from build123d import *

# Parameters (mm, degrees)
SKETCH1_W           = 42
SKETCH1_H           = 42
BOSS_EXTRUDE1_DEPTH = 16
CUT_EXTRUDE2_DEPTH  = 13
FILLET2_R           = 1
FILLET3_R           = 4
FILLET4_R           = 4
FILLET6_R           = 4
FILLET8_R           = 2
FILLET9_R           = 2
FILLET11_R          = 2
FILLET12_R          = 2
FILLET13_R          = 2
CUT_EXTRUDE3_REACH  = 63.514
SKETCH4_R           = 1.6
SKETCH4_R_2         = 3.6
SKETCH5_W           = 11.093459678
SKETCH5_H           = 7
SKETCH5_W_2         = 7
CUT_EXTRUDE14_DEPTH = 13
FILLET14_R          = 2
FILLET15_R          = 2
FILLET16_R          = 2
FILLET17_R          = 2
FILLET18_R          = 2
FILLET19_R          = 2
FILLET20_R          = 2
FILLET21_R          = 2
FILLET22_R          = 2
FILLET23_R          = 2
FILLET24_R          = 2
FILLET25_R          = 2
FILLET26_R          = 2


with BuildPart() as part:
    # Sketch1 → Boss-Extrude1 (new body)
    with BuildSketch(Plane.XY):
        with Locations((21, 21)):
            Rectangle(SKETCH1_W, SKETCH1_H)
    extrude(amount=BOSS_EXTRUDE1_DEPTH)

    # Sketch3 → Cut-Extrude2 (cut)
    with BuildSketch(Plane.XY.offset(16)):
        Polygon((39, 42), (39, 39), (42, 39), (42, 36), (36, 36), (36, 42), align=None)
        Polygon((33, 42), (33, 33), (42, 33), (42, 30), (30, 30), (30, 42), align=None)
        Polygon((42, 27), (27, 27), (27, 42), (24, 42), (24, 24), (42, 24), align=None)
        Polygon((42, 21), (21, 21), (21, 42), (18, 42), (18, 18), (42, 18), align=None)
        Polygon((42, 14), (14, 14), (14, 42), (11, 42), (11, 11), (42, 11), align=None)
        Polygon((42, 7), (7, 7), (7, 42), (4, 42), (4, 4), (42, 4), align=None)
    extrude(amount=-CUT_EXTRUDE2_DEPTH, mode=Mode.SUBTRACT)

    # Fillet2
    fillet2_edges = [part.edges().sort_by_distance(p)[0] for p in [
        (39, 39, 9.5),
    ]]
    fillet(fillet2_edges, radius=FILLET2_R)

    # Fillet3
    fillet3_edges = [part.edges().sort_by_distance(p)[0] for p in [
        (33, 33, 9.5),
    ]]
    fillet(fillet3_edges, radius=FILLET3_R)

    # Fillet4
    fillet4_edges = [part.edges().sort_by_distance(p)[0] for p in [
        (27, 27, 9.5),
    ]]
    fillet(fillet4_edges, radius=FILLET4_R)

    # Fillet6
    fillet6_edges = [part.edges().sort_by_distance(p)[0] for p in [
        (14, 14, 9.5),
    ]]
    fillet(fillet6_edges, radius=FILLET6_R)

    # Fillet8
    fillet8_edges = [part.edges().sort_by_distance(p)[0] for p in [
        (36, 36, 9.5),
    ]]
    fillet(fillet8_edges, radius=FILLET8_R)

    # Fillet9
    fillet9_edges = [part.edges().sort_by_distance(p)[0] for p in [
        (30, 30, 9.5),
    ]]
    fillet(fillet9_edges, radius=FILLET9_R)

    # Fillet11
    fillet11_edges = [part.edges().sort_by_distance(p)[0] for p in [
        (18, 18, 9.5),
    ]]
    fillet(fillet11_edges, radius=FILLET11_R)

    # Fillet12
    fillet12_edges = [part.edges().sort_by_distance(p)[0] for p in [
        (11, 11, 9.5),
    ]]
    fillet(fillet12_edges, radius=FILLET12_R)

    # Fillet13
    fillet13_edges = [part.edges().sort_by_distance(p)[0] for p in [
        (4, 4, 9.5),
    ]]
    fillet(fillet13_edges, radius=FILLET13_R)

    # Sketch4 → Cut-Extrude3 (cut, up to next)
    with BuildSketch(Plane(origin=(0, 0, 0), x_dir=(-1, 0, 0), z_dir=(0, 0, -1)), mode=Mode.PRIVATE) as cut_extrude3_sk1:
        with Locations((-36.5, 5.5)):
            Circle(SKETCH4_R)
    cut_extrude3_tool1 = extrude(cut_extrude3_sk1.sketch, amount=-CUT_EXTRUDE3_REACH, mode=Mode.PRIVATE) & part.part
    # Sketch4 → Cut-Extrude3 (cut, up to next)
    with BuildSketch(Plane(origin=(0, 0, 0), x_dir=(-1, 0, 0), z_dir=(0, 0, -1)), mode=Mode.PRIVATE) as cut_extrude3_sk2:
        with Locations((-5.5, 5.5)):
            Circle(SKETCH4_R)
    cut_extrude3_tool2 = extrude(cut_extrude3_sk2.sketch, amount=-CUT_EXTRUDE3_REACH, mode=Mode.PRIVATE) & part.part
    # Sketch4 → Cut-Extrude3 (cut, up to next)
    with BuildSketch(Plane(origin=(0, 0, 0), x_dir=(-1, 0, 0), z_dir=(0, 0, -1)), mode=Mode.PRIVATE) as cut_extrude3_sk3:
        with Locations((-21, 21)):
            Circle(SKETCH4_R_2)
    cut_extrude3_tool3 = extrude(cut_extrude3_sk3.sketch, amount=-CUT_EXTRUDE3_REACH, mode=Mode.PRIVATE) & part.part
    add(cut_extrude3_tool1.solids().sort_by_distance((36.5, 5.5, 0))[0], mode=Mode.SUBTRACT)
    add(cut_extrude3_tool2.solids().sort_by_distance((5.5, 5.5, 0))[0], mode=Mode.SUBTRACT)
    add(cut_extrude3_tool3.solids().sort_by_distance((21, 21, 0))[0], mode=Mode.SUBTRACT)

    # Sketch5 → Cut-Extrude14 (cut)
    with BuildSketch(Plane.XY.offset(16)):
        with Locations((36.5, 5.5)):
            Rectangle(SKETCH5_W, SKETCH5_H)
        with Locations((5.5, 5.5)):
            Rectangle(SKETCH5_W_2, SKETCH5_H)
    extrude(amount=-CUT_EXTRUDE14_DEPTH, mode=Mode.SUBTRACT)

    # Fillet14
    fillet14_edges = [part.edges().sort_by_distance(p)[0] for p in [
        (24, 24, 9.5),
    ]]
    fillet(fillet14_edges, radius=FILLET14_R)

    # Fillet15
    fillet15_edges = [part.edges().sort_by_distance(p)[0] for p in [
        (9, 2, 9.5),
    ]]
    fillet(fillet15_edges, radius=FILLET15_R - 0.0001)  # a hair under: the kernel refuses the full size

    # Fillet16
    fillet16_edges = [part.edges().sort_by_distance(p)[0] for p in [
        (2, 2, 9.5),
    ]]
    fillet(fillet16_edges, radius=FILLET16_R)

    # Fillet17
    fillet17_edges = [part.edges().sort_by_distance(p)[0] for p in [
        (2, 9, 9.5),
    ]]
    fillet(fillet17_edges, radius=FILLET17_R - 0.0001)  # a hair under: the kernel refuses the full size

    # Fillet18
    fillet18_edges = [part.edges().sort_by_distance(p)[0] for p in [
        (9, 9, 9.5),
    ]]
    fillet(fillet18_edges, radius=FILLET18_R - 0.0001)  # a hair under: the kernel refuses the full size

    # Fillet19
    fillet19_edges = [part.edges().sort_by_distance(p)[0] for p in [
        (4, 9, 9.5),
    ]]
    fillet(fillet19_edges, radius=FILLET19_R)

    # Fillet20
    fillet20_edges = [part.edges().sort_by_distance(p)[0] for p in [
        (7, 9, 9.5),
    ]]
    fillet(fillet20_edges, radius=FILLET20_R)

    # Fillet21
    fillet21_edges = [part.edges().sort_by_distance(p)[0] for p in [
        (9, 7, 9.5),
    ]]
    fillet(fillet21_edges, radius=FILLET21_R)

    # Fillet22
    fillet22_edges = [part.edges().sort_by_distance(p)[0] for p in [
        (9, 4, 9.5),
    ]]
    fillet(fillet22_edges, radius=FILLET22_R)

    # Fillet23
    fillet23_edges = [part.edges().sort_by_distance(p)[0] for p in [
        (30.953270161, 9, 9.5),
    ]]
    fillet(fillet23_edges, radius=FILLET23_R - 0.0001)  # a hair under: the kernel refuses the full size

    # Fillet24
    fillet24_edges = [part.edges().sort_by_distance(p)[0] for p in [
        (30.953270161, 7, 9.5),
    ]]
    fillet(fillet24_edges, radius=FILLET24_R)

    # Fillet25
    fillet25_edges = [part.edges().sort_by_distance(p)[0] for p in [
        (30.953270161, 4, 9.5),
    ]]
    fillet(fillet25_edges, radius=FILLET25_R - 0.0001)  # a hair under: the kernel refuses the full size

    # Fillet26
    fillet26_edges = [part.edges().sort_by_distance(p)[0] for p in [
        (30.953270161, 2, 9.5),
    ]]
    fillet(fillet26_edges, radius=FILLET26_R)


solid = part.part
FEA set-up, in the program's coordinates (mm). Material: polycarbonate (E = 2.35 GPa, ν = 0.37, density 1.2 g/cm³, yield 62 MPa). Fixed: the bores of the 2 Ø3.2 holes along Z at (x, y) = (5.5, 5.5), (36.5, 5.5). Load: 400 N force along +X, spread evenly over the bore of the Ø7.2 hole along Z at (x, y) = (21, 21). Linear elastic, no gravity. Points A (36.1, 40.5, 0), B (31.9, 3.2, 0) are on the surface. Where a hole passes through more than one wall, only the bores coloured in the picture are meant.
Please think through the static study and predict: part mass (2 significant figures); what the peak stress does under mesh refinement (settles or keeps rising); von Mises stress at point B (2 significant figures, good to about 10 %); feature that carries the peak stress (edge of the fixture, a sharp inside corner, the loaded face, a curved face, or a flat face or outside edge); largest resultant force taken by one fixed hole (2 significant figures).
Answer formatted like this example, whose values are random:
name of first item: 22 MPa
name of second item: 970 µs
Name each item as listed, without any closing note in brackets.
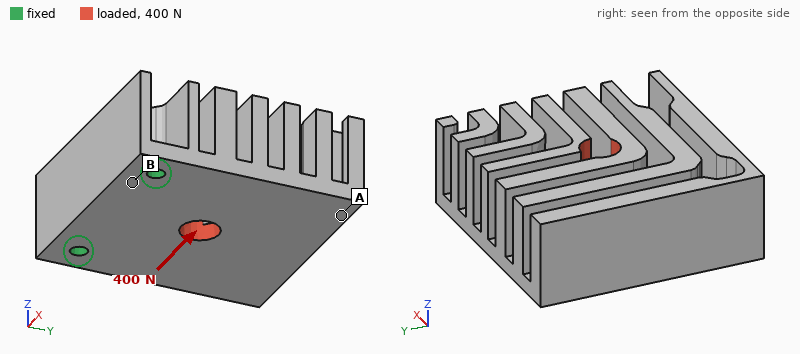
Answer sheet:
part mass: 21 g
what the peak stress does under mesh refinement: keeps rising
von Mises stress at point B: 2.7 MPa
feature that carries the peak stress: edge of the fixture
largest resultant force taken by one fixed hole: 290 N
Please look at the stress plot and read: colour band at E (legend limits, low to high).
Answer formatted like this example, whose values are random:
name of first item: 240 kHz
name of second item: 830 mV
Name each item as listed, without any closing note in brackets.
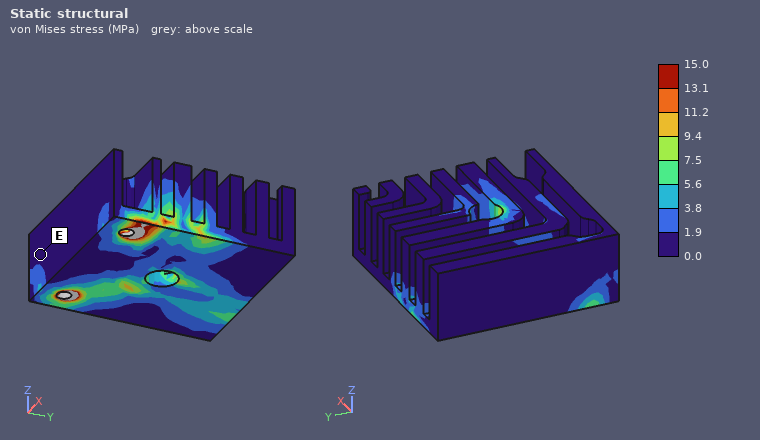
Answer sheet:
colour band at E: 0.0 to 1.9 MPa
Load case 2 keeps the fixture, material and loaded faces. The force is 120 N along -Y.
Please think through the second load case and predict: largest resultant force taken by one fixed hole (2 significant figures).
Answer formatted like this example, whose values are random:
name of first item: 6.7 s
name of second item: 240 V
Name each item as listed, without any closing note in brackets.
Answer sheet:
largest resultant force taken by one fixed hole: 63 N
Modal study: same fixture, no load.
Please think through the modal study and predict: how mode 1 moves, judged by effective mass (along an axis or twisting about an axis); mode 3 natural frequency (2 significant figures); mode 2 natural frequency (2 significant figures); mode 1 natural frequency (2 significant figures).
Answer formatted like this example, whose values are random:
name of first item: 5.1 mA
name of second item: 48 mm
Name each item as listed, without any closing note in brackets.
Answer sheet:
how mode 1 moves, judged by effective mass: along Z
mode 3 natural frequency: 1600 Hz
mode 2 natural frequency: 930 Hz
mode 1 natural frequency: 410 Hz
